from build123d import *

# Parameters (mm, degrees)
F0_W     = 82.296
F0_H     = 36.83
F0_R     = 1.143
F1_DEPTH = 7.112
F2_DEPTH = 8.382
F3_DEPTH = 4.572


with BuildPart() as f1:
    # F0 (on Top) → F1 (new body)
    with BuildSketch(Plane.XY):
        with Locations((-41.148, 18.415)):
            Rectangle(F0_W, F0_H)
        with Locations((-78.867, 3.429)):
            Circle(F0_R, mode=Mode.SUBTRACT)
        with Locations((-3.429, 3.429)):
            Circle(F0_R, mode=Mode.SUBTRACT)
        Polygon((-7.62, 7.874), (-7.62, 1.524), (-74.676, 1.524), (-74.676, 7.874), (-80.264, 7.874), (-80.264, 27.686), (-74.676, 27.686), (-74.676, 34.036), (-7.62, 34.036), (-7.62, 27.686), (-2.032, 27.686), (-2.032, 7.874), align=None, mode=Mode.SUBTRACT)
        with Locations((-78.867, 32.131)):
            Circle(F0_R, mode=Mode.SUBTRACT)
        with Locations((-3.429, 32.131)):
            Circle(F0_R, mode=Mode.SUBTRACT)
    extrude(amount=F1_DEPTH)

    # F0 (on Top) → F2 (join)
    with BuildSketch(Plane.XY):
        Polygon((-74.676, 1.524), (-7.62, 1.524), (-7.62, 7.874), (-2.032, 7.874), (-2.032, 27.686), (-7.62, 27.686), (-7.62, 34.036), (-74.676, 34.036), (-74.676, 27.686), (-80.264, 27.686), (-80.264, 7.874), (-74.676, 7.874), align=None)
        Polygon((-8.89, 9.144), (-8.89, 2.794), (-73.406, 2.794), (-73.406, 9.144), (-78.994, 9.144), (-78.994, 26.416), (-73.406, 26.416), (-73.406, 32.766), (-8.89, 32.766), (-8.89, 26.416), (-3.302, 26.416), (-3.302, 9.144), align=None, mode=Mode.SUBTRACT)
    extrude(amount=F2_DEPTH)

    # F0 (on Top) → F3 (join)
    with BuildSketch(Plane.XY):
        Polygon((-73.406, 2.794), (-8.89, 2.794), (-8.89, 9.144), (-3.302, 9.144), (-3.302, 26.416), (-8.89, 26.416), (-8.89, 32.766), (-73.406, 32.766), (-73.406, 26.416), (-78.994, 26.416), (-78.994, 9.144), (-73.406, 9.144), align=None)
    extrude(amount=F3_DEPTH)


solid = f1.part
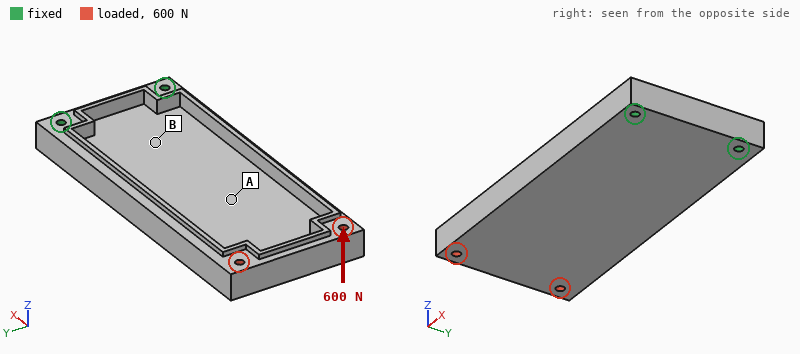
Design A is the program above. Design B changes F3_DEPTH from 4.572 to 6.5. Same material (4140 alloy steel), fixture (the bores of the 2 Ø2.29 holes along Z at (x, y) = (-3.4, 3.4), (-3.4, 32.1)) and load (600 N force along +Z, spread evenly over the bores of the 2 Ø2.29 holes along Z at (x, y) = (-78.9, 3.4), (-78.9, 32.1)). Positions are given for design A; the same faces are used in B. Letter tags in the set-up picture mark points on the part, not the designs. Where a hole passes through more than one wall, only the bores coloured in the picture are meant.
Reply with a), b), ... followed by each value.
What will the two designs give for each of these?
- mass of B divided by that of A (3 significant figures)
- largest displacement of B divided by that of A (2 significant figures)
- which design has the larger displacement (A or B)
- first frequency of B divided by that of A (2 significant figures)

a) 1.25
b) 0.66
c) A
d) 1.1
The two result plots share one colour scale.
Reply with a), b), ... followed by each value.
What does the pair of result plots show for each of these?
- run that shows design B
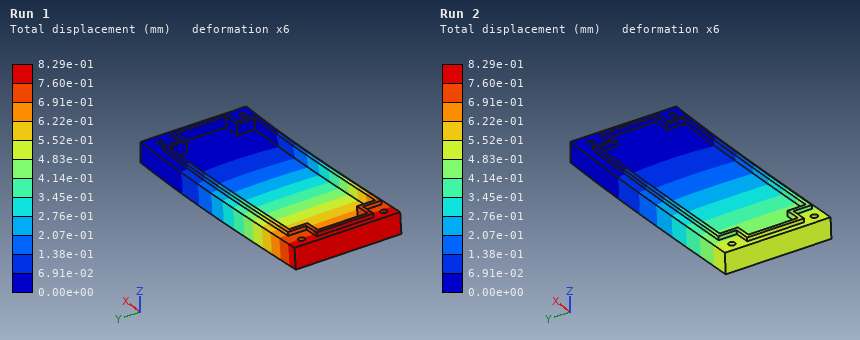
a) Run 2
